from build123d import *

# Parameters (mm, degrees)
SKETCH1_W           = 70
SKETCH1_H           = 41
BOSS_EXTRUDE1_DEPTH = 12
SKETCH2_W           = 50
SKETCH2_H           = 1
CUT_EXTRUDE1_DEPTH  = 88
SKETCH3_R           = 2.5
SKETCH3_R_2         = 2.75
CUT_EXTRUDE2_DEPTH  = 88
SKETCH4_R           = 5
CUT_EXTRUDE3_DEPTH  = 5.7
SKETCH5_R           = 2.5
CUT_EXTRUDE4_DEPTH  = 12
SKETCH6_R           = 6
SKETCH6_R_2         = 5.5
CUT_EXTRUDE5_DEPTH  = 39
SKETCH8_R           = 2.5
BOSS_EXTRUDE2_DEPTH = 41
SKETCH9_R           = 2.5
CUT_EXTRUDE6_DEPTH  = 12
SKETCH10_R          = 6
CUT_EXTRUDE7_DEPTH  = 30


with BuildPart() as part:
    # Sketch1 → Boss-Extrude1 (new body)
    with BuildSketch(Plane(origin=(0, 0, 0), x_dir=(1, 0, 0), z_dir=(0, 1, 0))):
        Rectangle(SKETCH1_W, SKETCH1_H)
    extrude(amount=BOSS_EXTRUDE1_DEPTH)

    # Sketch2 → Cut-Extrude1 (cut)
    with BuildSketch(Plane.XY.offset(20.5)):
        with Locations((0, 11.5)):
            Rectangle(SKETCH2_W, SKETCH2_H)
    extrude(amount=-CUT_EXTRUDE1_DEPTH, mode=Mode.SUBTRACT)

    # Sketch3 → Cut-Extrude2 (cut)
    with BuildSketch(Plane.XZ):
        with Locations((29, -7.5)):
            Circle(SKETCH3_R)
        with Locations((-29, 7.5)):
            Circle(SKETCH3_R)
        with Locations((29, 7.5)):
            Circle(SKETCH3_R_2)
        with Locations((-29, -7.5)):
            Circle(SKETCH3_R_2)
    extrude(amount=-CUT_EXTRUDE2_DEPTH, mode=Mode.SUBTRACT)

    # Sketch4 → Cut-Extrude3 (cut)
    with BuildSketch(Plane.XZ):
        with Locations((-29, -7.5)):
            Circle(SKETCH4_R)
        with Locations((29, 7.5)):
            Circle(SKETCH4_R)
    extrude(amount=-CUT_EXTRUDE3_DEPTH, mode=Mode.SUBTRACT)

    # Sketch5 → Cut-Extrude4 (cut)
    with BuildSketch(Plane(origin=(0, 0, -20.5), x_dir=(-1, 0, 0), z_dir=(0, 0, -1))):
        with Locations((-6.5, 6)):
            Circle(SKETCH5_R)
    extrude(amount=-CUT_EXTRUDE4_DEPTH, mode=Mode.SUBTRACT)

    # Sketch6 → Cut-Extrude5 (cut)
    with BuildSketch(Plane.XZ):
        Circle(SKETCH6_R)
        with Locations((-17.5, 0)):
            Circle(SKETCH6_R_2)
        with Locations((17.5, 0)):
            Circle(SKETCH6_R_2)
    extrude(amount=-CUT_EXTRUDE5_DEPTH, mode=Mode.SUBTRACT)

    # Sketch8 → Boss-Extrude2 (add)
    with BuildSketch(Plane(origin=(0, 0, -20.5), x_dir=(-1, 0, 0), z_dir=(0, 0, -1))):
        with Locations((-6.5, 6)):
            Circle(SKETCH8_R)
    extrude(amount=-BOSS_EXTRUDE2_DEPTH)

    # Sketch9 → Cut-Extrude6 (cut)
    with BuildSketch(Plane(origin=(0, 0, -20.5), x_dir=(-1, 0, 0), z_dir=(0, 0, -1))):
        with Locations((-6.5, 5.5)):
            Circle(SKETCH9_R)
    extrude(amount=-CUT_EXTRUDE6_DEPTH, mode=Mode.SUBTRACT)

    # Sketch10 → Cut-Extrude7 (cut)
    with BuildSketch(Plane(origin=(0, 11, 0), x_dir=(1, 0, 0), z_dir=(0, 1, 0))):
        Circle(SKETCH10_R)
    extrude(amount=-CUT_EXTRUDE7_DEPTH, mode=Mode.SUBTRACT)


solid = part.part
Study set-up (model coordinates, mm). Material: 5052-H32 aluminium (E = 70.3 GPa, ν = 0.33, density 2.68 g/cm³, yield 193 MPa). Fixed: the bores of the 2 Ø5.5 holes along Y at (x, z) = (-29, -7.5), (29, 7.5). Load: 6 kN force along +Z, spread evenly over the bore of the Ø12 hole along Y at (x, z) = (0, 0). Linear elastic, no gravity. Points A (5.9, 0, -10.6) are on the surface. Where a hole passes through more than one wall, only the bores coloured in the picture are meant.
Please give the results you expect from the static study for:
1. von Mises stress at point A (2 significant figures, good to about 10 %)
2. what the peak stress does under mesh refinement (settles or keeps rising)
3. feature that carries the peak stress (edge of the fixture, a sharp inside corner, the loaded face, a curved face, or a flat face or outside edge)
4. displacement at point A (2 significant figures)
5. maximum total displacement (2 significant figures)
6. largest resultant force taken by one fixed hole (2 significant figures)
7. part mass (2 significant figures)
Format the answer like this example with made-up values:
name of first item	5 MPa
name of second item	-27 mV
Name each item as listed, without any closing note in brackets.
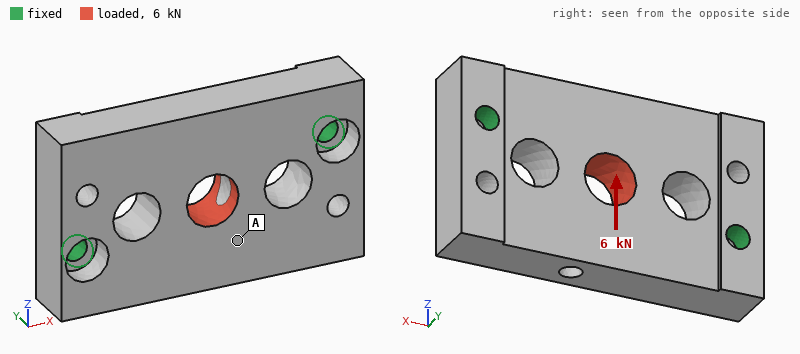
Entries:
von Mises stress at point A	13 MPa
what the peak stress does under mesh refinement	keeps rising
feature that carries the peak stress	edge of the fixture
displacement at point A	30 µm
maximum total displacement	36 µm
largest resultant force taken by one fixed hole	3.1 kN
part mass	73 g
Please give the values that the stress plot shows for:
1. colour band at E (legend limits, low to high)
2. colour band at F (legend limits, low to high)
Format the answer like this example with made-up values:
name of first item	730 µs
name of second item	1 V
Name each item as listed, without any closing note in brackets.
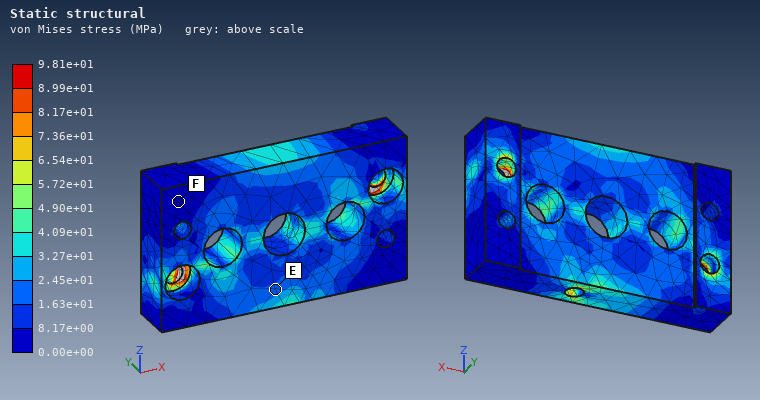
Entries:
colour band at E	1.63e+01 to 2.45e+01 MPa
colour band at F	0.00e+00 to 8.17e+00 MPa
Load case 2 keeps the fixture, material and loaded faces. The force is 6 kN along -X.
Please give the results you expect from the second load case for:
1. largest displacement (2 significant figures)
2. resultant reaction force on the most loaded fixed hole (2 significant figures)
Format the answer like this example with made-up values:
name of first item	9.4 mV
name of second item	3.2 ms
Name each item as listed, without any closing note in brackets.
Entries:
largest displacement	14 µm
resultant reaction force on the most loaded fixed hole	3.0 kN
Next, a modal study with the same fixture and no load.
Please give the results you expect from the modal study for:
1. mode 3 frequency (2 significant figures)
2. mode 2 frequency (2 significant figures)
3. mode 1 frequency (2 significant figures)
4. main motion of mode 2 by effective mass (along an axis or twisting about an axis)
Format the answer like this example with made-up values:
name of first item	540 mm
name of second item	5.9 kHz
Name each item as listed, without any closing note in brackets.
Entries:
mode 3 frequency	12 kHz
mode 2 frequency	7600 Hz
mode 1 frequency	5500 Hz
main motion of mode 2 by effective mass	along Y
